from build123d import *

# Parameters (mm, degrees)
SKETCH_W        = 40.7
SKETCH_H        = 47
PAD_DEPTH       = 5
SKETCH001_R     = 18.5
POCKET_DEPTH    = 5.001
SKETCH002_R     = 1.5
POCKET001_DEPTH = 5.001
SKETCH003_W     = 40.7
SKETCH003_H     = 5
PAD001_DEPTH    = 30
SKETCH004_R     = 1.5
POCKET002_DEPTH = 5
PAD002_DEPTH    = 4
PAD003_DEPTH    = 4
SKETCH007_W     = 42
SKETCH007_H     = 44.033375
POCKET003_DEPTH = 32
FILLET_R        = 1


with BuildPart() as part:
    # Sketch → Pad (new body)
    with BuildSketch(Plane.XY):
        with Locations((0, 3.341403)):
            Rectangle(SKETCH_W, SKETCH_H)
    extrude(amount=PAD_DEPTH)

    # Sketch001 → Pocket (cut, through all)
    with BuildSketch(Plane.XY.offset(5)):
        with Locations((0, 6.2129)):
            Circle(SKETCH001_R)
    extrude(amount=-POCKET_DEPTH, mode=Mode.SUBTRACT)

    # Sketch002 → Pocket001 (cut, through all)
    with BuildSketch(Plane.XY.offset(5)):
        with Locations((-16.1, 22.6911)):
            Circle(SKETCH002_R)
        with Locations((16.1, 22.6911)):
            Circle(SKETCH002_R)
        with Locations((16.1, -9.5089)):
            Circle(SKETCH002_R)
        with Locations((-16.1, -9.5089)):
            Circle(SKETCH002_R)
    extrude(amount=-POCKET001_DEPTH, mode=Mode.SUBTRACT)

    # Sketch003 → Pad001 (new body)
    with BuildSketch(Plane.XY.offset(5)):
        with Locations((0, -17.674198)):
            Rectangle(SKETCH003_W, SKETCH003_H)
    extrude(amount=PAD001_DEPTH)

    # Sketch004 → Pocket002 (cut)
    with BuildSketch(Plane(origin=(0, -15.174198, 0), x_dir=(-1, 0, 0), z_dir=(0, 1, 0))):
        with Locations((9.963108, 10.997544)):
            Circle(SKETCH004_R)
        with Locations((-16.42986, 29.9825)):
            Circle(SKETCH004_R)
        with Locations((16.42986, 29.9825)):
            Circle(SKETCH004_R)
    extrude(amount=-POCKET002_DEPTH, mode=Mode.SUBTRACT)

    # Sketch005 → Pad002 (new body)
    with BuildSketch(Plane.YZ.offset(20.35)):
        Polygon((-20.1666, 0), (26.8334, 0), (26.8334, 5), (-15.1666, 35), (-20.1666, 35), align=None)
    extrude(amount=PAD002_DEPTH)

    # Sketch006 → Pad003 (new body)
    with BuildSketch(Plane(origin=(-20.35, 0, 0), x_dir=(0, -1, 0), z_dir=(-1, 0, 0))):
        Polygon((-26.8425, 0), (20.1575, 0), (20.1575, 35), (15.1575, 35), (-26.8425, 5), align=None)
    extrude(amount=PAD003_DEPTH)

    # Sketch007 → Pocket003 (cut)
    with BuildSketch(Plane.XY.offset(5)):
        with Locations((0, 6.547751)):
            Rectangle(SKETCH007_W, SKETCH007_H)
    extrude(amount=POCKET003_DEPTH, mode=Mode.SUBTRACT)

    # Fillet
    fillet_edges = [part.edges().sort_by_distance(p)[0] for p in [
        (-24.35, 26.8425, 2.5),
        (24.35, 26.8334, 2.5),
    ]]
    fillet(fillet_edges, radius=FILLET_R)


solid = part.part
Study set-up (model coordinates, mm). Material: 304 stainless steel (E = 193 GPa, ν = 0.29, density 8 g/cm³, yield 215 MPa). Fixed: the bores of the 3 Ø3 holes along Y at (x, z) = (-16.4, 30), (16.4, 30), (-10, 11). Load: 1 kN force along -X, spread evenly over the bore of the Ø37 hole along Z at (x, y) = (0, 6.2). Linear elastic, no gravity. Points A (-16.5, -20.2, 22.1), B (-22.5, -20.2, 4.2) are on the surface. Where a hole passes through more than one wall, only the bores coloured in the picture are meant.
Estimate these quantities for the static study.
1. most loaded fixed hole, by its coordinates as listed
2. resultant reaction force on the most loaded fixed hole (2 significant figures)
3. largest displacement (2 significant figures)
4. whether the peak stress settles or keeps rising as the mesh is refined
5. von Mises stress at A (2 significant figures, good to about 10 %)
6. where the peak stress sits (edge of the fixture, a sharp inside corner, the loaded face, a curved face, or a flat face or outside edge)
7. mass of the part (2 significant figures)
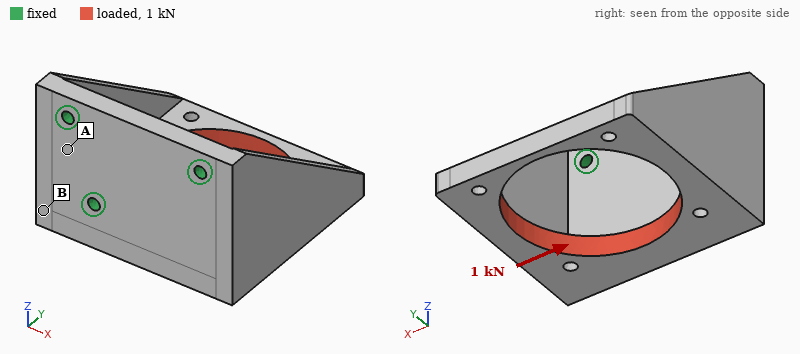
(-10, 11)
940 N
0.11 mm
keeps rising
36 MPa
edge of the fixture
140 g
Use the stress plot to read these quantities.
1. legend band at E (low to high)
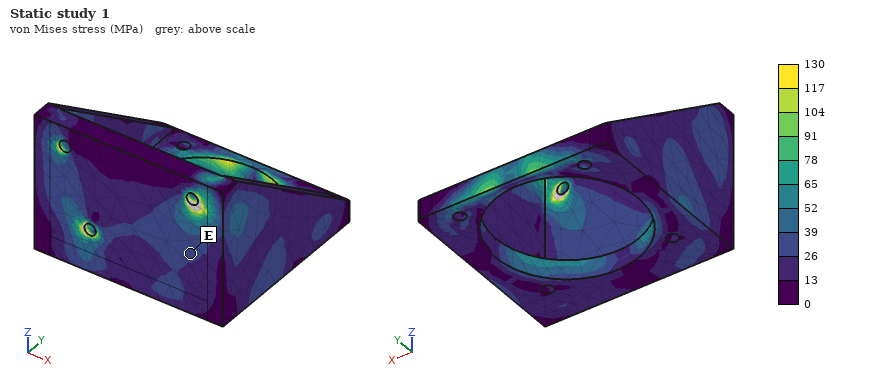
26 to 39 MPa
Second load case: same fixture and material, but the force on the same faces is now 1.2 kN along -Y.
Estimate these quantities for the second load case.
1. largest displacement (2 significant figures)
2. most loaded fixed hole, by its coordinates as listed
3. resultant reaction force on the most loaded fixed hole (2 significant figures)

65 µm
(-10, 11)
1.2 kN
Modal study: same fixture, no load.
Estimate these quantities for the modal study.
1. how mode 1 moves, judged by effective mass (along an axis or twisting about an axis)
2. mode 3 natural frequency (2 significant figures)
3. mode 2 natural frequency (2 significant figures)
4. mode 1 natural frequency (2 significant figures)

along X
6200 Hz
3900 Hz
2200 Hz
